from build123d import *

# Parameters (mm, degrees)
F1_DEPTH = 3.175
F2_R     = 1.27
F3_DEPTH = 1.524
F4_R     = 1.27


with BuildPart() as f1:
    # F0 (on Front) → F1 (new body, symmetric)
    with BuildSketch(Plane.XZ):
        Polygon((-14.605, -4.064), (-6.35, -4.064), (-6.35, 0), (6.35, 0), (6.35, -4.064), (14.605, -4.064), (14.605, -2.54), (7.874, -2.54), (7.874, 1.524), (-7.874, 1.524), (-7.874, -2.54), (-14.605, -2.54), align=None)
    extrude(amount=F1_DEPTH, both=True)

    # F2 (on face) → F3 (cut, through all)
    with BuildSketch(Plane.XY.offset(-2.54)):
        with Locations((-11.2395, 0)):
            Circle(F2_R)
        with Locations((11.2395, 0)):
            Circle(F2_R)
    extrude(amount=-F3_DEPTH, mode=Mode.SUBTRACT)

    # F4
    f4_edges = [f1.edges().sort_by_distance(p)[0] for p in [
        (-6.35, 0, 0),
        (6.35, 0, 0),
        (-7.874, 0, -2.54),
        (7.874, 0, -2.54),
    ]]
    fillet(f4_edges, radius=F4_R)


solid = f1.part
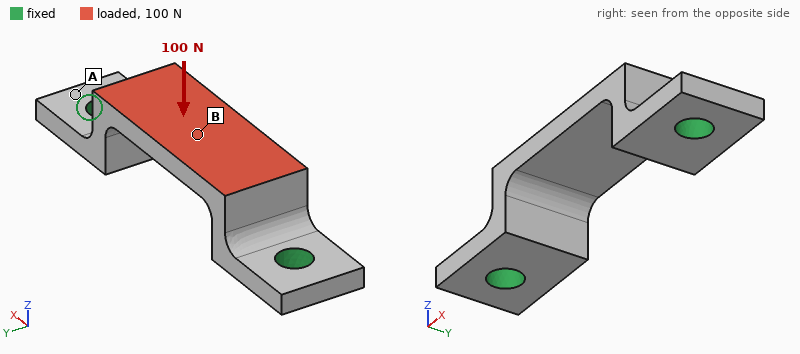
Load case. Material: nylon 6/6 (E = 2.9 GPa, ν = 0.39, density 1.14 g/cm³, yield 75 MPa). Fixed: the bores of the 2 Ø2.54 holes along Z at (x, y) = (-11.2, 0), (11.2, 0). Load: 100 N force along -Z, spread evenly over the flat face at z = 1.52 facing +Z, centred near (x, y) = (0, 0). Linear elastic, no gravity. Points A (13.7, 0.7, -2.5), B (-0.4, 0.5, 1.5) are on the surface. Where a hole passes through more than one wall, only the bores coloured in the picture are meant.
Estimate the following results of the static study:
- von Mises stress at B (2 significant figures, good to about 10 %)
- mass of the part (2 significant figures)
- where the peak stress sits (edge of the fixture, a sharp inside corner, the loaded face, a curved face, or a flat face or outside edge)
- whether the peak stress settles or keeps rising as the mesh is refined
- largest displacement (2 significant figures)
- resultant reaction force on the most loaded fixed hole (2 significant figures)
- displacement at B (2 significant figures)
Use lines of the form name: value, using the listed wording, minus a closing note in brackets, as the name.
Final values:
von Mises stress at B: 22 MPa
mass of the part: 0.40 g
where the peak stress sits: edge of the fixture
whether the peak stress settles or keeps rising as the mesh is refined: keeps rising
largest displacement: 0.16 mm
resultant reaction force on the most loaded fixed hole: 71 N
displacement at B: 0.15 mm
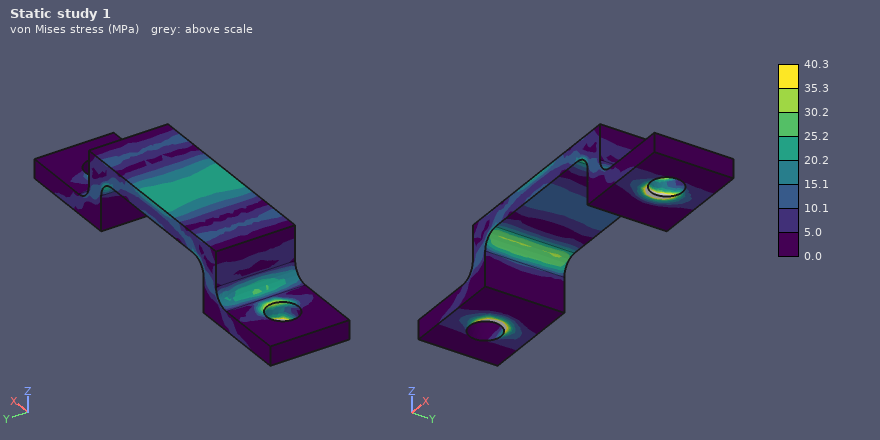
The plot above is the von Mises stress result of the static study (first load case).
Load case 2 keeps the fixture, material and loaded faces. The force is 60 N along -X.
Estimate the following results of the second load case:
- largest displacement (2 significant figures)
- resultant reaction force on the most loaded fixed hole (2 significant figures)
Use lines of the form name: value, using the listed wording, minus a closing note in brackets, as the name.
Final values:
largest displacement: 92 µm
resultant reaction force on the most loaded fixed hole: 32 N
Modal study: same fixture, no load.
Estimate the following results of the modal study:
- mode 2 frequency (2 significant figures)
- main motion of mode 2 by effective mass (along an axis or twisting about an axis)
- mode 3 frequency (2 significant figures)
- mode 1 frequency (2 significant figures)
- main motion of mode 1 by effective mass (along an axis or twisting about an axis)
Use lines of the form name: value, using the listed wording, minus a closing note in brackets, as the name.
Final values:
mode 2 frequency: 8500 Hz
main motion of mode 2 by effective mass: along X
mode 3 frequency: 11 kHz
mode 1 frequency: 6400 Hz
main motion of mode 1 by effective mass: along Y
